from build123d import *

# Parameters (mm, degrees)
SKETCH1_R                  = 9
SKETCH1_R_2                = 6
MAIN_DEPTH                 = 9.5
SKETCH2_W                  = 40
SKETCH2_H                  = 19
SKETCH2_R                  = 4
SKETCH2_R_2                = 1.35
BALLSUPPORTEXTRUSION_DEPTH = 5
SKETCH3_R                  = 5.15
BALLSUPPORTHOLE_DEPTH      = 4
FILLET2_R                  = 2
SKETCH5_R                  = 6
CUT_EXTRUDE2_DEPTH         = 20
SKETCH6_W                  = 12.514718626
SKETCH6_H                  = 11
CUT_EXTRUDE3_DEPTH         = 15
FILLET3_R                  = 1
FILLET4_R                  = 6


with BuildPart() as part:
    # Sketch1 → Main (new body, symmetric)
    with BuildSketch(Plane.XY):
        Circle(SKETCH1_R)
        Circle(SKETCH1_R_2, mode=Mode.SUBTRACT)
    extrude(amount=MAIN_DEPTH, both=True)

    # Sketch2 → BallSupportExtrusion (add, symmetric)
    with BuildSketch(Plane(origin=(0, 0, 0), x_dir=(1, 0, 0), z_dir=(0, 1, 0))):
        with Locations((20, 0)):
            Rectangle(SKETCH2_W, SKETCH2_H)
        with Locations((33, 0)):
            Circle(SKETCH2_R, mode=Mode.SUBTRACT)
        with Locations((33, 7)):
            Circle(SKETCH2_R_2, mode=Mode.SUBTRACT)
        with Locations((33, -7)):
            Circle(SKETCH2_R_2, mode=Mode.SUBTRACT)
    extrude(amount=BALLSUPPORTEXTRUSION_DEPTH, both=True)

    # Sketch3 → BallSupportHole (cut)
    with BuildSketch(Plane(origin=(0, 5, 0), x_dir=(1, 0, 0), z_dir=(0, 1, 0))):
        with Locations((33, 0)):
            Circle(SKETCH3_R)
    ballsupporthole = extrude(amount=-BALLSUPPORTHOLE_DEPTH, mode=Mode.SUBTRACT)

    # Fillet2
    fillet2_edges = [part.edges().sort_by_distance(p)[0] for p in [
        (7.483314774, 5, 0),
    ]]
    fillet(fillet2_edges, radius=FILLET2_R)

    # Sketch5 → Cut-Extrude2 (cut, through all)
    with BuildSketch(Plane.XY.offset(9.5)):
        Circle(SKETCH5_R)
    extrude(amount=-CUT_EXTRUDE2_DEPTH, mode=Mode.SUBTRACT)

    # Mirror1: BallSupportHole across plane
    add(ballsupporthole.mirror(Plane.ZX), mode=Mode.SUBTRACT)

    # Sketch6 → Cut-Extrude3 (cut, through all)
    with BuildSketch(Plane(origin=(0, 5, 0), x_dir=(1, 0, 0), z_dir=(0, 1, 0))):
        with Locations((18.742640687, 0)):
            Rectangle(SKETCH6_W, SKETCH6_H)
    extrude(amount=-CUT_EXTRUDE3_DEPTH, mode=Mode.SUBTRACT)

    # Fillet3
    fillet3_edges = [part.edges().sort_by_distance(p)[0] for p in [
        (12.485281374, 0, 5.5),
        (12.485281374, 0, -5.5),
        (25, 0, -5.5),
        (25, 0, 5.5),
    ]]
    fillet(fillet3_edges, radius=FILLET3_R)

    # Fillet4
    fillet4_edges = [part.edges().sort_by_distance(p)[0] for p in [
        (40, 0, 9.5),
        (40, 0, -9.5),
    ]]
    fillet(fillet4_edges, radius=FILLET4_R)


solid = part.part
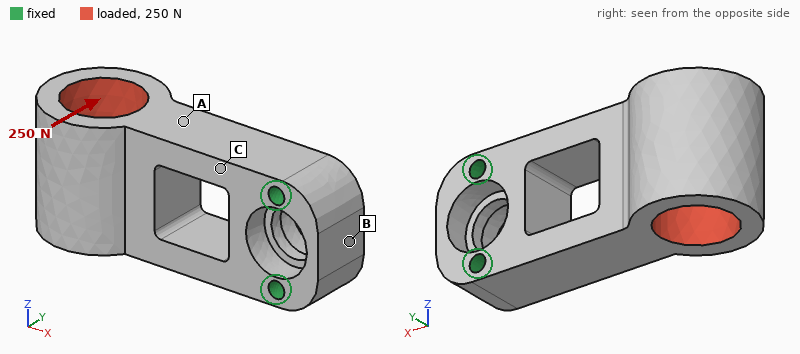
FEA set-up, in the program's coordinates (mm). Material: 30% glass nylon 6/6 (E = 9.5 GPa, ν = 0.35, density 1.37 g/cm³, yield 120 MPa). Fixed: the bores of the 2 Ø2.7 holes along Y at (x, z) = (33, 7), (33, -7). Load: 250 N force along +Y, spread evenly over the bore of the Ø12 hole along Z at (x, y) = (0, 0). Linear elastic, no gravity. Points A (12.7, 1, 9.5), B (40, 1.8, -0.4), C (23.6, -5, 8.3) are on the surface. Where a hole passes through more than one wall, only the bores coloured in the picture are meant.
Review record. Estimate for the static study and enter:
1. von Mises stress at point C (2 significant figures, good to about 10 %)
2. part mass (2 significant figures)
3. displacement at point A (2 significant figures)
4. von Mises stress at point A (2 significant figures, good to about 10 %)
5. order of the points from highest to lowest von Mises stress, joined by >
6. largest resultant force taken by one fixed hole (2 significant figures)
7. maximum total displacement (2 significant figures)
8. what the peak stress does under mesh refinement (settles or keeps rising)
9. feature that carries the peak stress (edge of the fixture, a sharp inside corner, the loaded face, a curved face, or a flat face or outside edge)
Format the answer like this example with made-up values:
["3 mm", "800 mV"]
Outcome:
["42 MPa", "8.6 g", "0.18 mm", "13 MPa", "C > A > B", "130 N", "0.64 mm", "keeps rising", "edge of the fixture"]
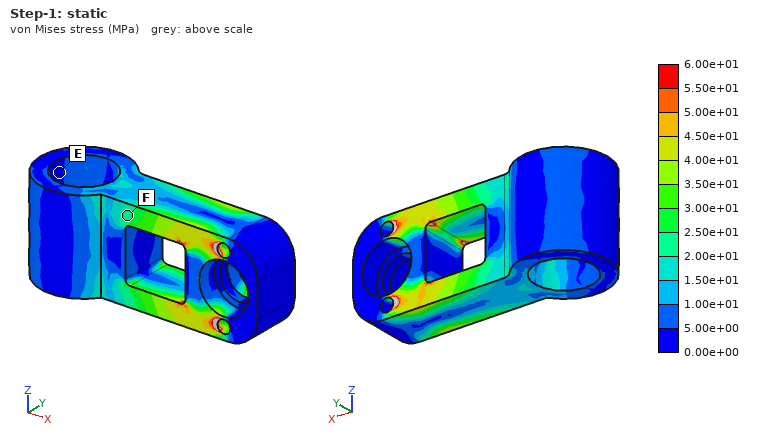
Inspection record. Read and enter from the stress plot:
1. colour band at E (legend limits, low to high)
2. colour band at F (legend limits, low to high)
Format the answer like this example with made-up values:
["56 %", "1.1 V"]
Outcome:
["0.00e+00 to 5.00e+00 MPa", "2.00e+01 to 2.50e+01 MPa"]
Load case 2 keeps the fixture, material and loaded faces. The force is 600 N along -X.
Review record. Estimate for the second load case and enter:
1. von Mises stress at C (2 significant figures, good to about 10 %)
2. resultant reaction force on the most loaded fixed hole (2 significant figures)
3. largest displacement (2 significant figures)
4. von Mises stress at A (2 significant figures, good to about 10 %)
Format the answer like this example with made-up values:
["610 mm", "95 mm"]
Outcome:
["7.0 MPa", "300 N", "46 µm", "3.8 MPa"]
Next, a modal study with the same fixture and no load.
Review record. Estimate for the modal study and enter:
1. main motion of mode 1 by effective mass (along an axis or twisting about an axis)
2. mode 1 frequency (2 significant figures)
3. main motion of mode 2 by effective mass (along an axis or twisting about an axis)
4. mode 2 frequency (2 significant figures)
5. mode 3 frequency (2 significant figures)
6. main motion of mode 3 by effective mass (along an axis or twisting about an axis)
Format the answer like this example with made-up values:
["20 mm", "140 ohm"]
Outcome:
["along Y", "1800 Hz", "along Z", "2700 Hz", "4900 Hz", "twisting about X"]
